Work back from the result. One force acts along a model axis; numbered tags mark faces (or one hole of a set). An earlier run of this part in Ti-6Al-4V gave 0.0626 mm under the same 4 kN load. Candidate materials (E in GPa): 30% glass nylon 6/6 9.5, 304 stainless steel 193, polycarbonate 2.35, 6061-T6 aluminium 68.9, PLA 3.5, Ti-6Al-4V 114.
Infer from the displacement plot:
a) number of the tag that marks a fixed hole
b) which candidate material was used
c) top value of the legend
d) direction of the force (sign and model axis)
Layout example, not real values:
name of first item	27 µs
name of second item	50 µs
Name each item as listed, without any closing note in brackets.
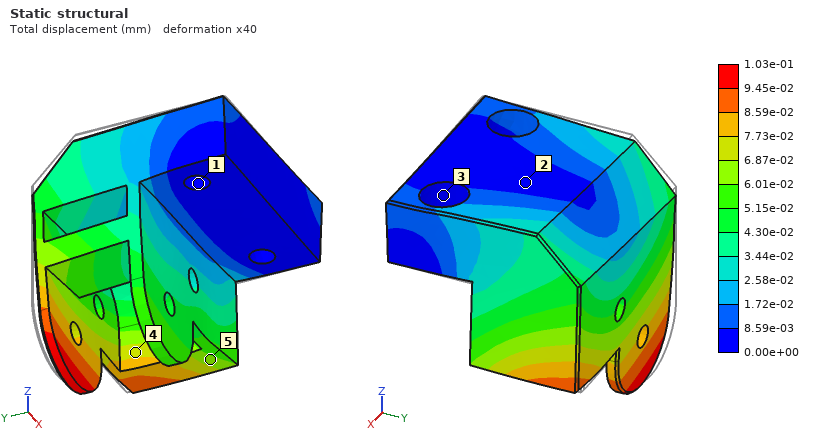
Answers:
number of the tag that marks a fixed hole	1
which candidate material was used	6061-T6 aluminium
top value of the legend	1.03e-01 mm
direction of the force	+X
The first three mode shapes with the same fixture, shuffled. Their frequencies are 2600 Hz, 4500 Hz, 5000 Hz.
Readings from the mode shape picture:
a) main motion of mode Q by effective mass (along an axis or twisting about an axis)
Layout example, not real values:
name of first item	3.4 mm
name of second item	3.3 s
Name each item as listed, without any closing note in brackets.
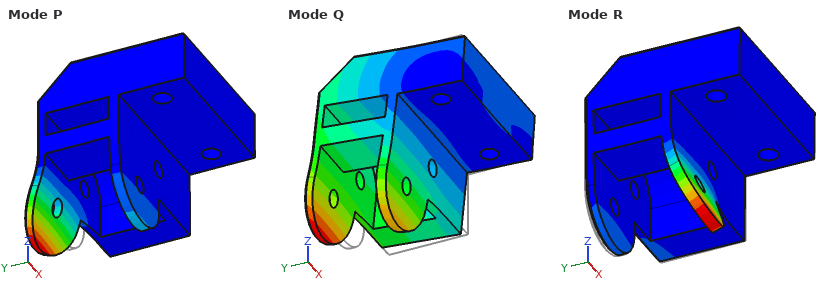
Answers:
main motion of mode Q by effective mass	along Z
